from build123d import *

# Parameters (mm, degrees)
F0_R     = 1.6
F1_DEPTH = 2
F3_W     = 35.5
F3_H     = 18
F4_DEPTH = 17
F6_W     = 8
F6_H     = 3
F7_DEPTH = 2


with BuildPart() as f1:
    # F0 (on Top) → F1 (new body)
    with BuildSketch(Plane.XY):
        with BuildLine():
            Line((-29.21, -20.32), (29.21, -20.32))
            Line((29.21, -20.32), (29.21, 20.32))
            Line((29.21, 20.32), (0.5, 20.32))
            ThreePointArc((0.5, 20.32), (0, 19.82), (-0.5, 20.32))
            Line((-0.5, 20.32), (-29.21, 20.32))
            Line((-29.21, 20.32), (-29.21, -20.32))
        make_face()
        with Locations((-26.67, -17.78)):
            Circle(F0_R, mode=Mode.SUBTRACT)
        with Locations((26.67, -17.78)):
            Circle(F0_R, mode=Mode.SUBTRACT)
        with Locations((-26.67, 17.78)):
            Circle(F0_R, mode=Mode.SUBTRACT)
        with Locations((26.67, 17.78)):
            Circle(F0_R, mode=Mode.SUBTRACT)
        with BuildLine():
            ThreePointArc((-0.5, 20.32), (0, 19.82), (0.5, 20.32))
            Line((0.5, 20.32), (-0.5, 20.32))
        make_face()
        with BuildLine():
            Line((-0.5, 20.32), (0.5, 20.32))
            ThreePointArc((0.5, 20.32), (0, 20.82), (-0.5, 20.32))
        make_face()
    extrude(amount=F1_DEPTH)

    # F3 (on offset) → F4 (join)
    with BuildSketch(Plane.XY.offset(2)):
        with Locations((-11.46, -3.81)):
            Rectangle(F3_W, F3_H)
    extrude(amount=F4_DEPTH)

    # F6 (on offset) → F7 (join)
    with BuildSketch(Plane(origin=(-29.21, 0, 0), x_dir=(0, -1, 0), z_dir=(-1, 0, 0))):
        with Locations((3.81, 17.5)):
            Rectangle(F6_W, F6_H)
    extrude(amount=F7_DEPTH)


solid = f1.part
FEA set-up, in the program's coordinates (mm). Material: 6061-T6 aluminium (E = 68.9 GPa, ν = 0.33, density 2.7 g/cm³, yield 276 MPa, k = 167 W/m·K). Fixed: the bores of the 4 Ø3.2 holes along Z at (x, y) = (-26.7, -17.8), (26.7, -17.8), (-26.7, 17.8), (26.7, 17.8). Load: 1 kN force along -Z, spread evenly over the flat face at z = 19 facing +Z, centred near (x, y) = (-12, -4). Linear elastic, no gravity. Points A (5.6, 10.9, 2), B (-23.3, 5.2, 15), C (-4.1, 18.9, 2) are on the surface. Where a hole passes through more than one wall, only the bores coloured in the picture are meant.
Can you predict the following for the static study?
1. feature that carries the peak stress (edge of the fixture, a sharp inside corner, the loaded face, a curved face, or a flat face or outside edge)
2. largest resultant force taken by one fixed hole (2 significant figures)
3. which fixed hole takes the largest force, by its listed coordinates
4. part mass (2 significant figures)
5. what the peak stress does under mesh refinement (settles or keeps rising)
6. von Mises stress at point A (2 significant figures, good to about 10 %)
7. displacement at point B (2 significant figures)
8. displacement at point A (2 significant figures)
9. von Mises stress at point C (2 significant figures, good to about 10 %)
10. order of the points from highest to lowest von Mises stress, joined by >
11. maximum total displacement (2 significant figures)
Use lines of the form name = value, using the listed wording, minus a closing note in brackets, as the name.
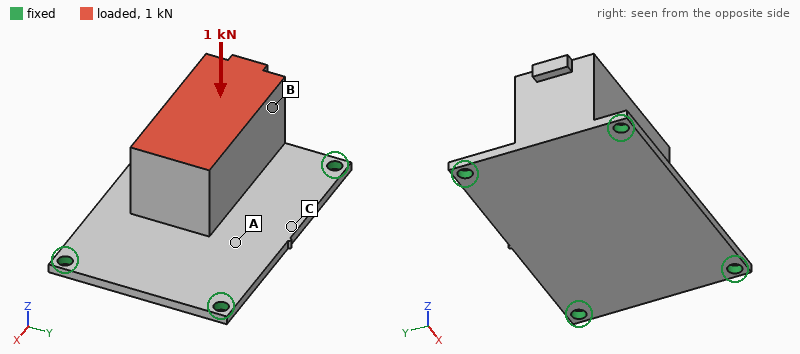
feature that carries the peak stress = edge of the fixture
largest resultant force taken by one fixed hole = 500 N
which fixed hole takes the largest force, by its listed coordinates = (-26.7, -17.8)
part mass = 42 g
what the peak stress does under mesh refinement = keeps rising
von Mises stress at point A = 74 MPa
displacement at point B = 0.095 mm
displacement at point A = 0.17 mm
von Mises stress at point C = 43 MPa
order of the points from highest to lowest von Mises stress, joined by > = A > C > B
maximum total displacement = 0.20 mm
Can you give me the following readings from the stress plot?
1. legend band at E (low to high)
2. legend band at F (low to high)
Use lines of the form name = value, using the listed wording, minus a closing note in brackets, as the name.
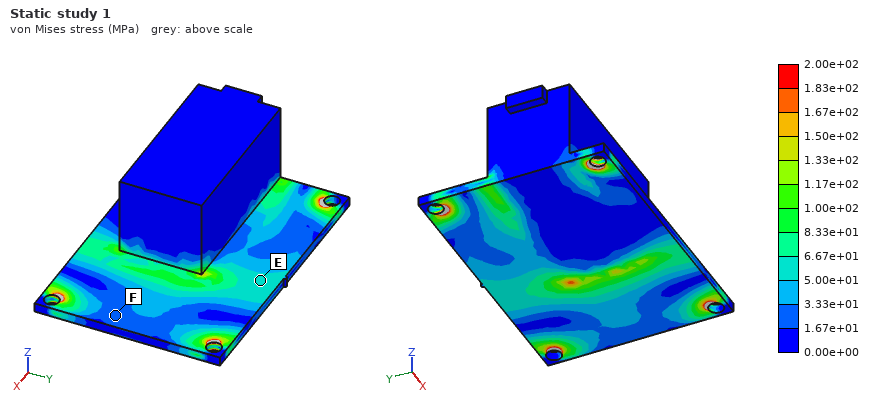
legend band at E = 5.00e+01 to 6.67e+01 MPa
legend band at F = 1.67e+01 to 3.33e+01 MPa
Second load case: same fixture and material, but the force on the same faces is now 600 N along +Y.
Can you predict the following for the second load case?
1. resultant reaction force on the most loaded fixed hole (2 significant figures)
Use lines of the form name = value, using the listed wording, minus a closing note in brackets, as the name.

resultant reaction force on the most loaded fixed hole = 420 N
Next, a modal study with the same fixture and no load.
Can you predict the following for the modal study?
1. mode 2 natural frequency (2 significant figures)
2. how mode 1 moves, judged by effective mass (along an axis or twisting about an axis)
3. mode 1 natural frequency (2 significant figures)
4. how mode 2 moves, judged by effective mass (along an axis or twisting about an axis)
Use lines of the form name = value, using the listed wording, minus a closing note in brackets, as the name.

mode 2 natural frequency = 3000 Hz
how mode 1 moves, judged by effective mass = along Z
mode 1 natural frequency = 2000 Hz
how mode 2 moves, judged by effective mass = along Y
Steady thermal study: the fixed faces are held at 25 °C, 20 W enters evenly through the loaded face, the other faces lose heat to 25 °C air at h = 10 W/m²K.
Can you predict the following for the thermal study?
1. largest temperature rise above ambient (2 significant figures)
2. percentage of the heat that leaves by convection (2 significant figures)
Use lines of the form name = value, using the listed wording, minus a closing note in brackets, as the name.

largest temperature rise above ambient = 19 K
percentage of the heat that leaves by convection = 3.8 %
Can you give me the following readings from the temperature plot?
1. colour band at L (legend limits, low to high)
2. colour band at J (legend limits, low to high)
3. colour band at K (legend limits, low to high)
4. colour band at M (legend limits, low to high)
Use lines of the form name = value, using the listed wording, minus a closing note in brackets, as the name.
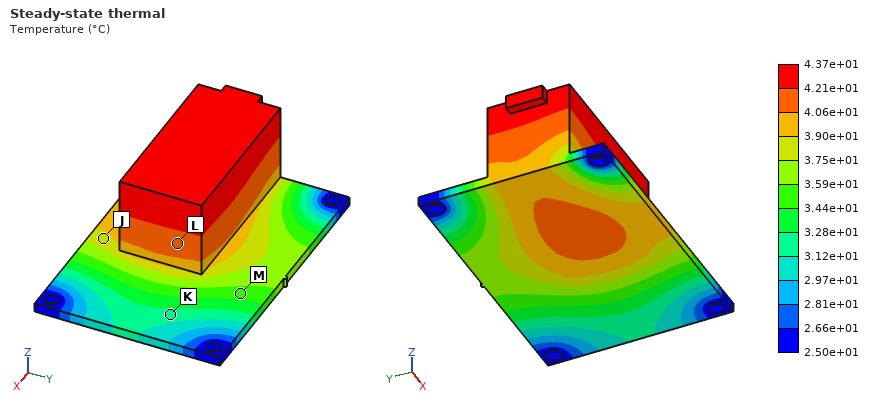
colour band at L = 4.06e+01 to 4.21e+01 °C
colour band at J = 3.75e+01 to 3.90e+01 °C
colour band at K = 3.12e+01 to 3.28e+01 °C
colour band at M = 3.44e+01 to 3.59e+01 °C
